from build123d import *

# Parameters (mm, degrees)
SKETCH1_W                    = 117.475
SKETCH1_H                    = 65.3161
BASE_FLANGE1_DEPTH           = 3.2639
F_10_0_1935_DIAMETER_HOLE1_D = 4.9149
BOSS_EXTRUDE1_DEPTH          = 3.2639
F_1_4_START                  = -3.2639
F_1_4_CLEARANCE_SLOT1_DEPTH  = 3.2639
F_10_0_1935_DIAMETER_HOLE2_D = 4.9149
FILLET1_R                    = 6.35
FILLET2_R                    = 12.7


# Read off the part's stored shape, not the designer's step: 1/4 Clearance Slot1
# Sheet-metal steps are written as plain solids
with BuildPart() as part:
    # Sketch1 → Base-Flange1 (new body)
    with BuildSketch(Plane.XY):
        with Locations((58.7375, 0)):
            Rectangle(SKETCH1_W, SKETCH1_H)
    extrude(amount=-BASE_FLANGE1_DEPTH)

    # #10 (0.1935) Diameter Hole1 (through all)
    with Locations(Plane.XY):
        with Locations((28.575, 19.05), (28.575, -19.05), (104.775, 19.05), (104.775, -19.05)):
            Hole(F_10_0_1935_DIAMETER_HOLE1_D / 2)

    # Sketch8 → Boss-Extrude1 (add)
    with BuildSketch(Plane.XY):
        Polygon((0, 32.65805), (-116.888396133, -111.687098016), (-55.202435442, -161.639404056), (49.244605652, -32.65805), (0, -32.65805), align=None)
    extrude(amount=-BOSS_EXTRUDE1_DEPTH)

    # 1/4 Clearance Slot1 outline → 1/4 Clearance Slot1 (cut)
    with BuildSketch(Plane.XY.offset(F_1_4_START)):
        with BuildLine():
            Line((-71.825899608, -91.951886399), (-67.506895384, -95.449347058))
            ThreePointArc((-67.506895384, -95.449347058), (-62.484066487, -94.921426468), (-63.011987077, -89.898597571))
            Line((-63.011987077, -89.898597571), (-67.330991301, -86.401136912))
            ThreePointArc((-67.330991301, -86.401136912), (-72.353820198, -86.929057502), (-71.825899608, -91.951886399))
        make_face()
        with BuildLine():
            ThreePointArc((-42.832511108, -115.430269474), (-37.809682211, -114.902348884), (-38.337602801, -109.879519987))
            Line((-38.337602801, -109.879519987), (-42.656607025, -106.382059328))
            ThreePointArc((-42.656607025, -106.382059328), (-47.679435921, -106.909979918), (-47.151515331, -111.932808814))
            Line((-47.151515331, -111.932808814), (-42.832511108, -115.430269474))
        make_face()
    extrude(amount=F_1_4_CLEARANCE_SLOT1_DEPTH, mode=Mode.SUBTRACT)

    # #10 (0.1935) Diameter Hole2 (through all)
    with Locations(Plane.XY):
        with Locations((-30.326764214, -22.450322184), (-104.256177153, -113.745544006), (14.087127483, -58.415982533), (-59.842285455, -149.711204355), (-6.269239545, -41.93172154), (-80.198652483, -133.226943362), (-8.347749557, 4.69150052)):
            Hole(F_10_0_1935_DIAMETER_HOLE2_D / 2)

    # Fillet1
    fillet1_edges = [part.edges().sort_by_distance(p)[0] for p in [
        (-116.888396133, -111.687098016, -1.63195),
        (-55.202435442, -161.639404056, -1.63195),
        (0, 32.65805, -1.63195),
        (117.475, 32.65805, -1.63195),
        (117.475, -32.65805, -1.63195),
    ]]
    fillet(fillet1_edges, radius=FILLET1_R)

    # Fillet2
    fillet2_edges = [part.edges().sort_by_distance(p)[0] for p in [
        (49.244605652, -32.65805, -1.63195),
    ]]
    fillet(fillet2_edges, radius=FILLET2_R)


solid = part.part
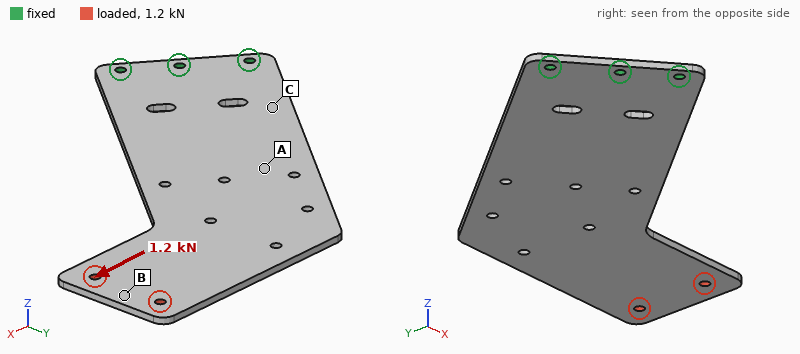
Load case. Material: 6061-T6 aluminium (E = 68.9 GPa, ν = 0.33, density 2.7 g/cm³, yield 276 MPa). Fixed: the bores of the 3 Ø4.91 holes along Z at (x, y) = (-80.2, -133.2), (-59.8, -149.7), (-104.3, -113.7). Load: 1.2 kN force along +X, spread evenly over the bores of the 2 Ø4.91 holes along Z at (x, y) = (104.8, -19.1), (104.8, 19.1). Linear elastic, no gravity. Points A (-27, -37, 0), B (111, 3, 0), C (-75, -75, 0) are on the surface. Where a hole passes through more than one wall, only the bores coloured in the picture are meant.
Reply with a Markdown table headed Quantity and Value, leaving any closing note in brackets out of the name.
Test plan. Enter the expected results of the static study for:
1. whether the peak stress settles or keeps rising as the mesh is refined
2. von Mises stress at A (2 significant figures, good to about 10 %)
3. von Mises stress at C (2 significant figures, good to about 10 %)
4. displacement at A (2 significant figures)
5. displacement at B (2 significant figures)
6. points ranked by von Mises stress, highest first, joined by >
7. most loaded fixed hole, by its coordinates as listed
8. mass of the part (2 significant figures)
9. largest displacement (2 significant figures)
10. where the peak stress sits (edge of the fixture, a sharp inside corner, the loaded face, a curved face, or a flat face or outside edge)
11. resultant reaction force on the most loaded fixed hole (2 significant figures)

| Quantity | Value |
|---|---|
| whether the peak stress settles or keeps rising as the mesh is refined | keeps rising |
| von Mises stress at A | 13 MPa |
| von Mises stress at C | 31 MPa |
| displacement at A | 0.12 mm |
| displacement at B | 0.34 mm |
| points ranked by von Mises stress, highest first, joined by > | C > A > B |
| most loaded fixed hole, by its coordinates as listed | (-104.3, -113.7) |
| mass of the part | 170 g |
| largest displacement | 0.37 mm |
| where the peak stress sits | edge of the fixture |
| resultant reaction force on the most loaded fixed hole | 3.0 kN |
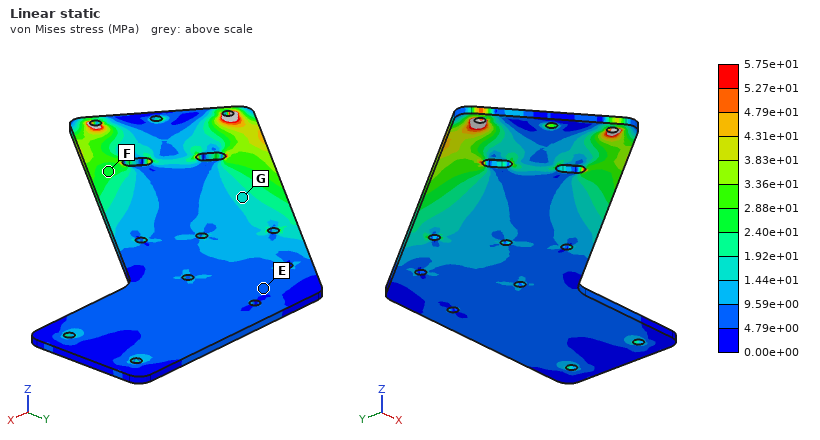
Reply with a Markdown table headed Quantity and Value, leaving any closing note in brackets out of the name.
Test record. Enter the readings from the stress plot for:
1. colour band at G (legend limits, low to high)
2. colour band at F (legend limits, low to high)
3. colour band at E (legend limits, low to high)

| Quantity | Value |
|---|---|
| colour band at G | 1.44e+01 to 1.92e+01 MPa |
| colour band at F | 2.40e+01 to 2.88e+01 MPa |
| colour band at E | 4.79e+00 to 9.59e+00 MPa |
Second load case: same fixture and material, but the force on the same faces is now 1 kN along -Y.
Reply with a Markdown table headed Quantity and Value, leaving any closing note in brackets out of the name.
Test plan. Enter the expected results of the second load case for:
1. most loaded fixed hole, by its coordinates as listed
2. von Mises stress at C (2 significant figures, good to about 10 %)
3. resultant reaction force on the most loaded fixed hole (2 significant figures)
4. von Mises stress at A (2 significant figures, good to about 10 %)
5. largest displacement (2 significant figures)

| Quantity | Value |
|---|---|
| most loaded fixed hole, by its coordinates as listed | (-59.8, -149.7) |
| von Mises stress at C | 35 MPa |
| resultant reaction force on the most loaded fixed hole | 3.3 kN |
| von Mises stress at A | 14 MPa |
| largest displacement | 0.57 mm |
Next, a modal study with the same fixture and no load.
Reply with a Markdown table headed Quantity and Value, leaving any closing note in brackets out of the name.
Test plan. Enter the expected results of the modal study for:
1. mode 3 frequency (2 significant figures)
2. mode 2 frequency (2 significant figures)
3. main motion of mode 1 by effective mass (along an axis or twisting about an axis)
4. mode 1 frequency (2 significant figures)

| Quantity | Value |
|---|---|
| mode 3 frequency | 360 Hz |
| mode 2 frequency | 200 Hz |
| main motion of mode 1 by effective mass | along Z |
| mode 1 frequency | 45 Hz |
